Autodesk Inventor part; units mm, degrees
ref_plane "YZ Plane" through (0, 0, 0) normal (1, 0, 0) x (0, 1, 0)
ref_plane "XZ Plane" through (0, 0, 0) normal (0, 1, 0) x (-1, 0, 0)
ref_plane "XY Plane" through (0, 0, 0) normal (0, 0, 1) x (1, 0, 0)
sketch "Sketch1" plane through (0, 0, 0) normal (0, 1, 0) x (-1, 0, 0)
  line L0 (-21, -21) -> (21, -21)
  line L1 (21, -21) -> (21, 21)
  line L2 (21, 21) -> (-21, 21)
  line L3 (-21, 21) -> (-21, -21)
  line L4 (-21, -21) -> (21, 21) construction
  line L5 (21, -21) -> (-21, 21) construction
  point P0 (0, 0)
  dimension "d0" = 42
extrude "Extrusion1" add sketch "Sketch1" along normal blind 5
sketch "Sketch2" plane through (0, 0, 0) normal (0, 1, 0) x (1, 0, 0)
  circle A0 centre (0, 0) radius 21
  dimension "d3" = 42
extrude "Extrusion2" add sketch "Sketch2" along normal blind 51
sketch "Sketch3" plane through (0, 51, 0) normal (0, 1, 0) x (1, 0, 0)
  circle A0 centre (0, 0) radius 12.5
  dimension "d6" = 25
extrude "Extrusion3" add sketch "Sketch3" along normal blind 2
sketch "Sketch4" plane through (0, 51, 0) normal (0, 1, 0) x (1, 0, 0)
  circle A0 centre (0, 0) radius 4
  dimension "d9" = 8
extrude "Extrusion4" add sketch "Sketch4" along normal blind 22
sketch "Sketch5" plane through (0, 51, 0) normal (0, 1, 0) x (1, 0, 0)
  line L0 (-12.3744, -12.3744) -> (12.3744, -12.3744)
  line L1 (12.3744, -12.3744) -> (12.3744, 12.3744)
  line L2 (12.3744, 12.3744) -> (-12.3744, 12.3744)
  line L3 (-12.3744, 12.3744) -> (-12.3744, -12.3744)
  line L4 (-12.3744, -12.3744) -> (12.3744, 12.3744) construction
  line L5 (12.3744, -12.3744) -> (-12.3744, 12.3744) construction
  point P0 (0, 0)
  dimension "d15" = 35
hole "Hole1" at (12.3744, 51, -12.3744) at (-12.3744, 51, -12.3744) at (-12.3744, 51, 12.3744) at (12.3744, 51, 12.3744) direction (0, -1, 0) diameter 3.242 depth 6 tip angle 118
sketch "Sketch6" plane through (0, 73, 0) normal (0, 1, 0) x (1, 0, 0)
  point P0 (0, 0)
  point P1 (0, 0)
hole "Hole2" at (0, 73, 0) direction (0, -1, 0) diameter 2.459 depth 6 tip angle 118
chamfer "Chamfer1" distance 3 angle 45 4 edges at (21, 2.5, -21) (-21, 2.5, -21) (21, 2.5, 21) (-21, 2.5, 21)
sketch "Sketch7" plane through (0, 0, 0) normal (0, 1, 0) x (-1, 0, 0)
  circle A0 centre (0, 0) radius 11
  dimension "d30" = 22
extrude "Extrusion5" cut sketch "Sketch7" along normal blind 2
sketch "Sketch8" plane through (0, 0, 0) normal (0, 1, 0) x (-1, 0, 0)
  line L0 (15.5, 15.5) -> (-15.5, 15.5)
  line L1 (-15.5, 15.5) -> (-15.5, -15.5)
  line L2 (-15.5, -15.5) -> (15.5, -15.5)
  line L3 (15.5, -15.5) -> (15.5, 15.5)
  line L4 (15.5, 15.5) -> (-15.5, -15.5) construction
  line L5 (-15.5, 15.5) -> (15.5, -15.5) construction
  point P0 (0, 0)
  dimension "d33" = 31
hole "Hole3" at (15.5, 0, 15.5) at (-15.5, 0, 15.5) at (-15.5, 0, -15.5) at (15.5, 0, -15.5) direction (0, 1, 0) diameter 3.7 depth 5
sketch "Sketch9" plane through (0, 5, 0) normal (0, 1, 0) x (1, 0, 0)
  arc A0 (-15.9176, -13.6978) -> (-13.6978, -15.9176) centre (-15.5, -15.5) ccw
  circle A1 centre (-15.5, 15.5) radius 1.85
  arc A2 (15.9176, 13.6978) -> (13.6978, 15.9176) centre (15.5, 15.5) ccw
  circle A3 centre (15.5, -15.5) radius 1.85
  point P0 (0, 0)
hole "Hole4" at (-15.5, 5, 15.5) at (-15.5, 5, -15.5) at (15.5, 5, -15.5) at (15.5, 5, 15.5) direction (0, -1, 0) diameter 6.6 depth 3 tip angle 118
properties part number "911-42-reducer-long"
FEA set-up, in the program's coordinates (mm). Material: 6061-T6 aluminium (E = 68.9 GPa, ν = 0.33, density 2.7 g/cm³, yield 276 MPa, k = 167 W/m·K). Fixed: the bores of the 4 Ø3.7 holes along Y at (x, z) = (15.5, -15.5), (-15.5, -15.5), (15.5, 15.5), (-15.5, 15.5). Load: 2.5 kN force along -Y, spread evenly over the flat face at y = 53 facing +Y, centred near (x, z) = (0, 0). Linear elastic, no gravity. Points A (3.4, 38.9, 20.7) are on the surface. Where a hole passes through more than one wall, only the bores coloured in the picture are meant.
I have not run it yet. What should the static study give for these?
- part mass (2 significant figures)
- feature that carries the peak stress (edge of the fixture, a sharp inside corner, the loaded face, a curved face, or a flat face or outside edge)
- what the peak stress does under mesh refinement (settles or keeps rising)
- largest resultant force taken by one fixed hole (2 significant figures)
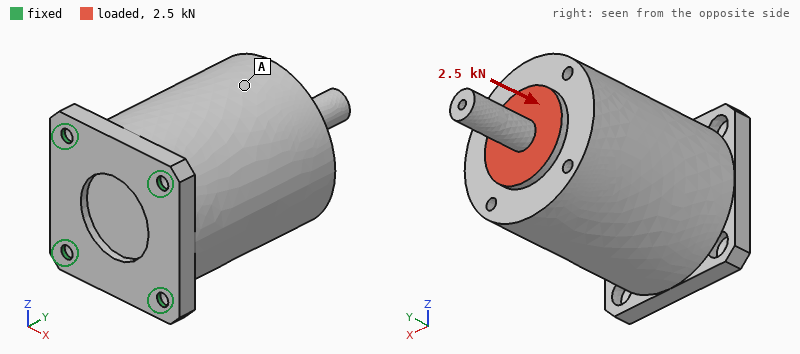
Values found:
200 g
edge of the fixture
keeps rising
710 N
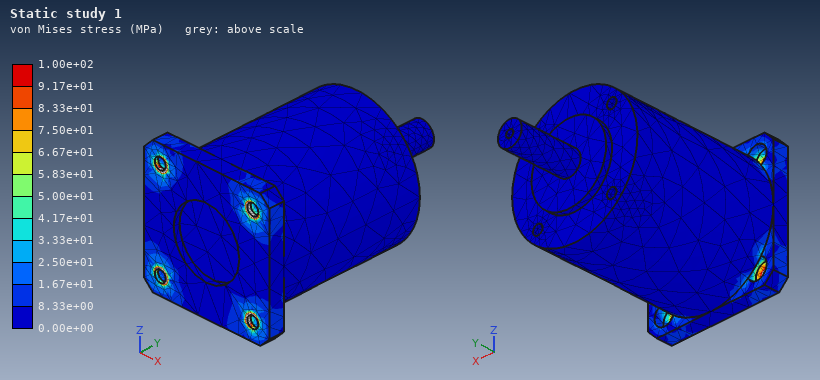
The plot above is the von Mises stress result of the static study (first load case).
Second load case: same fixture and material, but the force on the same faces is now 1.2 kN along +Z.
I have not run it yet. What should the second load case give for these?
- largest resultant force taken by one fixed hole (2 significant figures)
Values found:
1.1 kN
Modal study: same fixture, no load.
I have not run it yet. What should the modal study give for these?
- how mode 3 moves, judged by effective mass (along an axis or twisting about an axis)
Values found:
along Y
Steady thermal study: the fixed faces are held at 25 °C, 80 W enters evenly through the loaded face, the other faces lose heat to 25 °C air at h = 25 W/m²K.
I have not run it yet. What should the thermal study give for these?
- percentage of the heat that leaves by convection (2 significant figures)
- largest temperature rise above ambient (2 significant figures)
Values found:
8.0 %
38 K
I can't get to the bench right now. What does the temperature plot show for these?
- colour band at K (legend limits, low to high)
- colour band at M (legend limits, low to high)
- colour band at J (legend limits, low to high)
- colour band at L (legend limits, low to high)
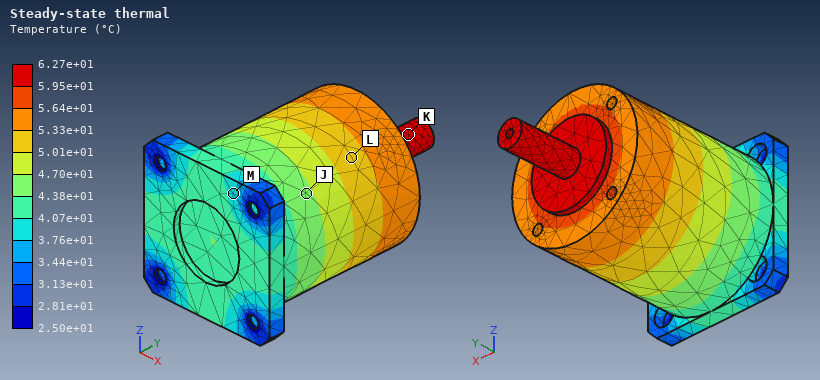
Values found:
5.95e+01 to 6.27e+01 °C
3.76e+01 to 4.07e+01 °C
4.38e+01 to 4.70e+01 °C
5.01e+01 to 5.33e+01 °C
